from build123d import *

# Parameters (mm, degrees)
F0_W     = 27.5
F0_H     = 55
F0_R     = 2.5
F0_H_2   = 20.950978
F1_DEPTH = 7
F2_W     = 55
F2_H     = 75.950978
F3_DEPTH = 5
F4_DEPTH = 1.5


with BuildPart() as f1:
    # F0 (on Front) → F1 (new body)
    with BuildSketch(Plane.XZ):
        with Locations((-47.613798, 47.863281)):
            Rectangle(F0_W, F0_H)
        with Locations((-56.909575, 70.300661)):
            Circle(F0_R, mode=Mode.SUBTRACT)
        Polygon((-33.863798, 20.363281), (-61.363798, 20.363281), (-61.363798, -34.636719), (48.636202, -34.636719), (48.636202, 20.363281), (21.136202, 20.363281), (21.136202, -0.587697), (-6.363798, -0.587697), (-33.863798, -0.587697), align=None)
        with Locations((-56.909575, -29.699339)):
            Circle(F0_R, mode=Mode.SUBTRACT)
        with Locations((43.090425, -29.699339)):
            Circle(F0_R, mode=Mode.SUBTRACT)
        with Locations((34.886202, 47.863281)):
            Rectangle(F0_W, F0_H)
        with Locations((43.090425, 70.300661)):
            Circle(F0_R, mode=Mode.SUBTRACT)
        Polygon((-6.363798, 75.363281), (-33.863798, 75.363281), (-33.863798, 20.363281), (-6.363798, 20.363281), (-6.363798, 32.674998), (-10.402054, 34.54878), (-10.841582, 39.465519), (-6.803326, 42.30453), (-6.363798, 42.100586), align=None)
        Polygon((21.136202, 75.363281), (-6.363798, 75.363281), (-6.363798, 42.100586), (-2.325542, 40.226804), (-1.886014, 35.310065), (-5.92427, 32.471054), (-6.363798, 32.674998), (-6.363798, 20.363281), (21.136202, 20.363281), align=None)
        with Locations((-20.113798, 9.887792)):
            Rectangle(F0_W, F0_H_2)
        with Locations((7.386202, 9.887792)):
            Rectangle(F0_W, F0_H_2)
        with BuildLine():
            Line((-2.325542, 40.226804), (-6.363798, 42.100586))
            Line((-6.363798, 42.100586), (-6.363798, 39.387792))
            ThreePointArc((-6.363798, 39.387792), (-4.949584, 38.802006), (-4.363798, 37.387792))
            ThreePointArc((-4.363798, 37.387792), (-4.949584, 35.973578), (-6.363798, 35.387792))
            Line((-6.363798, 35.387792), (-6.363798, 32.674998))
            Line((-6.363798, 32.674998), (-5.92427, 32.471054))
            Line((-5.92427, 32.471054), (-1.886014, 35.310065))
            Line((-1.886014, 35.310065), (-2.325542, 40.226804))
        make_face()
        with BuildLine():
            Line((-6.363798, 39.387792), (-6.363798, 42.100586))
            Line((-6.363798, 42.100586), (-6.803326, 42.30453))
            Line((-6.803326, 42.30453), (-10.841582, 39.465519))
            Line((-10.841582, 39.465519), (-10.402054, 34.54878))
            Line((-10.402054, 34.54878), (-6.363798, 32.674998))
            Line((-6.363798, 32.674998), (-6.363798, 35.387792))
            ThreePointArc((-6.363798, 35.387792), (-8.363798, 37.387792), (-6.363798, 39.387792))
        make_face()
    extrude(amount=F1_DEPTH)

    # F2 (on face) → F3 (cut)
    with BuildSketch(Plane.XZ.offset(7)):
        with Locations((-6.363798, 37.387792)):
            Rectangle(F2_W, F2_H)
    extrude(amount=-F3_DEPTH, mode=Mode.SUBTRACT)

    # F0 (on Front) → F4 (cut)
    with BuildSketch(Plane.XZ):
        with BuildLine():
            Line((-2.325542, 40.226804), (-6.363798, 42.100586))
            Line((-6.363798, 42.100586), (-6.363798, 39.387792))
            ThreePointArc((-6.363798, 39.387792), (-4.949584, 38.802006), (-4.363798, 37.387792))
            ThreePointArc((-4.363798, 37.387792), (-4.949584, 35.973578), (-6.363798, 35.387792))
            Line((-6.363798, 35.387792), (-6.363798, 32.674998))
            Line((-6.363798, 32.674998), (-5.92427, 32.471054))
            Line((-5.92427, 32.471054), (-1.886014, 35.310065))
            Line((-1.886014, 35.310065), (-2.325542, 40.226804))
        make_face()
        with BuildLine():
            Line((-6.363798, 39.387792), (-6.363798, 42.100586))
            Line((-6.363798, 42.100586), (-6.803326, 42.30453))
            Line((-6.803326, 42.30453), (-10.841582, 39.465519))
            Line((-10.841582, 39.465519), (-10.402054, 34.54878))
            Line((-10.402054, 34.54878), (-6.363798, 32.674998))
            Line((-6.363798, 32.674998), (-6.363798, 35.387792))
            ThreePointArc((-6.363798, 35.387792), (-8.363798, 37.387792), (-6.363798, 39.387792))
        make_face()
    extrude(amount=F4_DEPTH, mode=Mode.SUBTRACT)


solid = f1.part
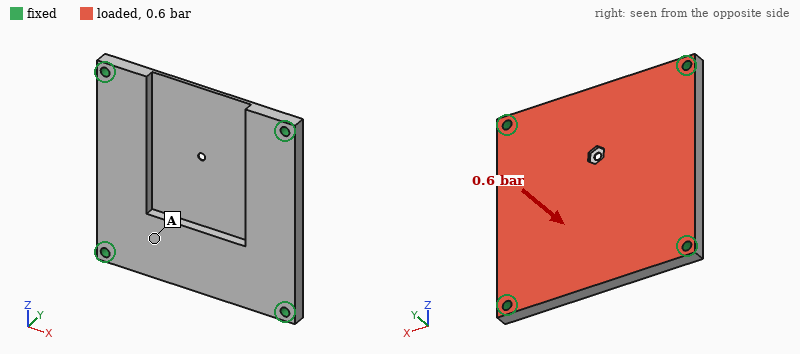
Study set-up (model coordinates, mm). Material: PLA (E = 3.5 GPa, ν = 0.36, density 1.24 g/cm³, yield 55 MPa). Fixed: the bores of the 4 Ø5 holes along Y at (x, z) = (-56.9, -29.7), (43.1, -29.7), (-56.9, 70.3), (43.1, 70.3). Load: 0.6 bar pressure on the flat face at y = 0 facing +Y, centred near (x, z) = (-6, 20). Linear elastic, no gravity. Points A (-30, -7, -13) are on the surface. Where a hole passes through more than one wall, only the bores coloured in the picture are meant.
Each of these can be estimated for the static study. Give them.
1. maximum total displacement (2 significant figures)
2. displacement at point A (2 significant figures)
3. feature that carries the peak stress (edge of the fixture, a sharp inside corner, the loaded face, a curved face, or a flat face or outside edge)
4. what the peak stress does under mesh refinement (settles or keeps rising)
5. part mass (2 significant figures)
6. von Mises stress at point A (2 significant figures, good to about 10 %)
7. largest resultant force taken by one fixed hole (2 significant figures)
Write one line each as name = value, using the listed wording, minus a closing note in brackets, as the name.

maximum total displacement = 1.3 mm
displacement at point A = 0.40 mm
feature that carries the peak stress = edge of the fixture
what the peak stress does under mesh refinement = keeps rising
part mass = 78 g
von Mises stress at point A = 4.2 MPa
largest resultant force taken by one fixed hole = 340 N
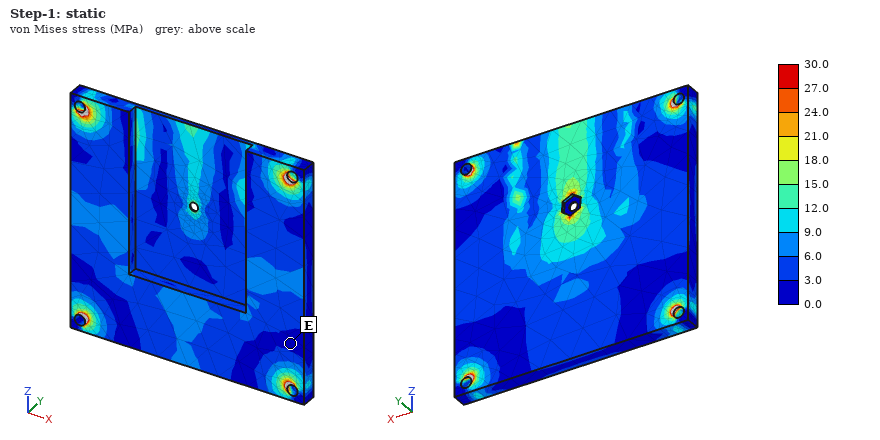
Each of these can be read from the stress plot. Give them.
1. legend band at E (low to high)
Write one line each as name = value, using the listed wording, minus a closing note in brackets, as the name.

legend band at E = 0.0 to 3.0 MPa
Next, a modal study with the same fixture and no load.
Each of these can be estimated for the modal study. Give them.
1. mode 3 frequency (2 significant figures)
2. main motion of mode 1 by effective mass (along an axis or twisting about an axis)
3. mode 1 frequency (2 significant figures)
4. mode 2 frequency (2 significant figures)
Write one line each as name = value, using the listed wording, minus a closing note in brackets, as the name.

mode 3 frequency = 1100 Hz
main motion of mode 1 by effective mass = along Y
mode 1 frequency = 750 Hz
mode 2 frequency = 1100 Hz
